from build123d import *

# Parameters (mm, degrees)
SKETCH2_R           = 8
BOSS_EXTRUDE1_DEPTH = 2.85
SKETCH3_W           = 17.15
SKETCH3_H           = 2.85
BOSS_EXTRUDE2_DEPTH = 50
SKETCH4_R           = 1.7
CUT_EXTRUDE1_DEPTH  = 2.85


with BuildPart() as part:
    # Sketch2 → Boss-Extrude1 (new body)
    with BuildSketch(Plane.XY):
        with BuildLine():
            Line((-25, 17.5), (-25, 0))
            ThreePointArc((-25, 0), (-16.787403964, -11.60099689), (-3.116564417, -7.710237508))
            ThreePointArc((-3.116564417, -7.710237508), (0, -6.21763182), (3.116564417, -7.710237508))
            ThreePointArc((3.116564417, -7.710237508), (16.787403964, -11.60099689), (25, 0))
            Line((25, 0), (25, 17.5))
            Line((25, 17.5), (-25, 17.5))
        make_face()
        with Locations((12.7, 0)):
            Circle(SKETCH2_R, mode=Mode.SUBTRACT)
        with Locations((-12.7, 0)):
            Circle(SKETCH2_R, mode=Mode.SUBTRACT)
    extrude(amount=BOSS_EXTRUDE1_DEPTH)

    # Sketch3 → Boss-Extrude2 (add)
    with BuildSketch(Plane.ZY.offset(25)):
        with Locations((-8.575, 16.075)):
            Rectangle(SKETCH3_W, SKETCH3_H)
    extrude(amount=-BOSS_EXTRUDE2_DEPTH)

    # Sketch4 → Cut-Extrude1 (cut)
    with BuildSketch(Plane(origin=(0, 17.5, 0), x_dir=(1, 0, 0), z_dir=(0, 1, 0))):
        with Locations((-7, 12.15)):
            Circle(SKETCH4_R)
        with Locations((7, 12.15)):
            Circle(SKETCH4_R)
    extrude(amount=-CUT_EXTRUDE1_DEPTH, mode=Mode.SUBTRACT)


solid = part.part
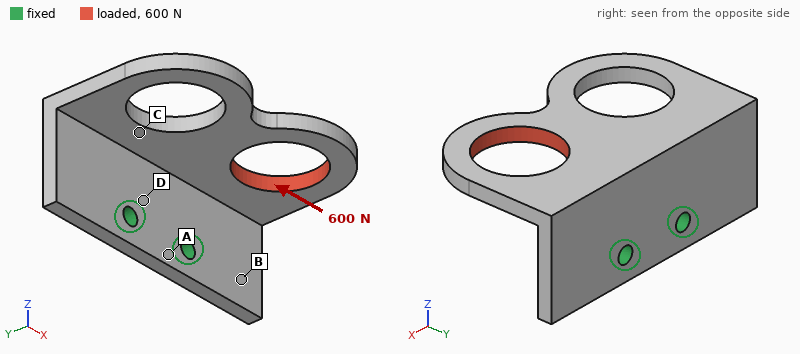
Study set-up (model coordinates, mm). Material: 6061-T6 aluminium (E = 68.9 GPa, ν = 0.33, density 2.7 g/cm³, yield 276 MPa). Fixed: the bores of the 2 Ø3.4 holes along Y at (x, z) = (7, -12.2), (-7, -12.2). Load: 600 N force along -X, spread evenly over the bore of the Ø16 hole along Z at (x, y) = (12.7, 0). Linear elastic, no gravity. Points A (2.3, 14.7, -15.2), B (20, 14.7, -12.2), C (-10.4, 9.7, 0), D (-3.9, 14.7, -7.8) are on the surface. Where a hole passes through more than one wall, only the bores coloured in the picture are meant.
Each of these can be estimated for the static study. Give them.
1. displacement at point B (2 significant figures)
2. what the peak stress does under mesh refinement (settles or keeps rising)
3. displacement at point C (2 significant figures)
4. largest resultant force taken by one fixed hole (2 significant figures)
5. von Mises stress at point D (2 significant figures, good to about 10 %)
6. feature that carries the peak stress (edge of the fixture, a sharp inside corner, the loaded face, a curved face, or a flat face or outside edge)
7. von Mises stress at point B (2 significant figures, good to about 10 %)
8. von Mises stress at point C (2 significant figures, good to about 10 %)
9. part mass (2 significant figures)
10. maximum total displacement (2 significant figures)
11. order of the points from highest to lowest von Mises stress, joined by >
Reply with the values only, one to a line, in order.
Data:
0.050 mm
keeps rising
0.091 mm
720 N
92 MPa
edge of the fixture
33 MPa
65 MPa
14 g
0.28 mm
D > C > B > A
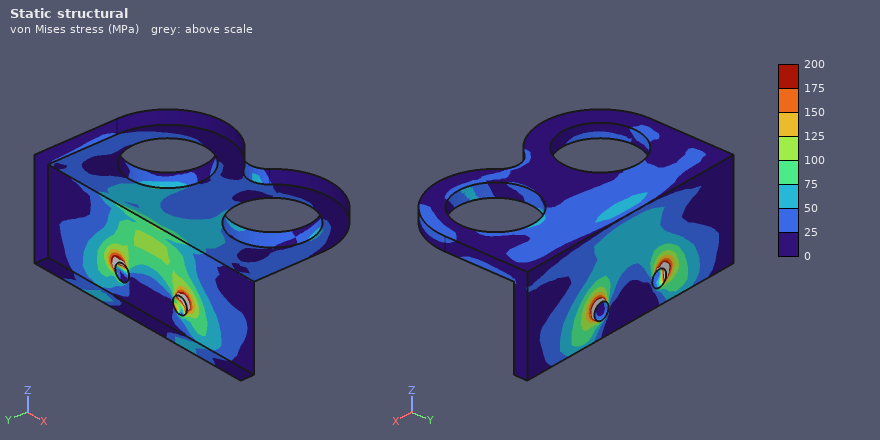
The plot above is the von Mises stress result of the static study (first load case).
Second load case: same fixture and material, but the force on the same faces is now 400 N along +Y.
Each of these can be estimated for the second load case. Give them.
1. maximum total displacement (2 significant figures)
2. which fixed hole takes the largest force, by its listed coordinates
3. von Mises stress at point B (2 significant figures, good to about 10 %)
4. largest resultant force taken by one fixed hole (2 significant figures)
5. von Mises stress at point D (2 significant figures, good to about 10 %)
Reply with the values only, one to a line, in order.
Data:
0.30 mm
(7, -12.2)
37 MPa
440 N
62 MPa
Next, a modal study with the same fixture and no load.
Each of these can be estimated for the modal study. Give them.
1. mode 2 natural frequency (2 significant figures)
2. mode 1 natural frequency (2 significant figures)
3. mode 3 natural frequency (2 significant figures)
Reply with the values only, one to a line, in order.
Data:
2900 Hz
2100 Hz
4700 Hz
